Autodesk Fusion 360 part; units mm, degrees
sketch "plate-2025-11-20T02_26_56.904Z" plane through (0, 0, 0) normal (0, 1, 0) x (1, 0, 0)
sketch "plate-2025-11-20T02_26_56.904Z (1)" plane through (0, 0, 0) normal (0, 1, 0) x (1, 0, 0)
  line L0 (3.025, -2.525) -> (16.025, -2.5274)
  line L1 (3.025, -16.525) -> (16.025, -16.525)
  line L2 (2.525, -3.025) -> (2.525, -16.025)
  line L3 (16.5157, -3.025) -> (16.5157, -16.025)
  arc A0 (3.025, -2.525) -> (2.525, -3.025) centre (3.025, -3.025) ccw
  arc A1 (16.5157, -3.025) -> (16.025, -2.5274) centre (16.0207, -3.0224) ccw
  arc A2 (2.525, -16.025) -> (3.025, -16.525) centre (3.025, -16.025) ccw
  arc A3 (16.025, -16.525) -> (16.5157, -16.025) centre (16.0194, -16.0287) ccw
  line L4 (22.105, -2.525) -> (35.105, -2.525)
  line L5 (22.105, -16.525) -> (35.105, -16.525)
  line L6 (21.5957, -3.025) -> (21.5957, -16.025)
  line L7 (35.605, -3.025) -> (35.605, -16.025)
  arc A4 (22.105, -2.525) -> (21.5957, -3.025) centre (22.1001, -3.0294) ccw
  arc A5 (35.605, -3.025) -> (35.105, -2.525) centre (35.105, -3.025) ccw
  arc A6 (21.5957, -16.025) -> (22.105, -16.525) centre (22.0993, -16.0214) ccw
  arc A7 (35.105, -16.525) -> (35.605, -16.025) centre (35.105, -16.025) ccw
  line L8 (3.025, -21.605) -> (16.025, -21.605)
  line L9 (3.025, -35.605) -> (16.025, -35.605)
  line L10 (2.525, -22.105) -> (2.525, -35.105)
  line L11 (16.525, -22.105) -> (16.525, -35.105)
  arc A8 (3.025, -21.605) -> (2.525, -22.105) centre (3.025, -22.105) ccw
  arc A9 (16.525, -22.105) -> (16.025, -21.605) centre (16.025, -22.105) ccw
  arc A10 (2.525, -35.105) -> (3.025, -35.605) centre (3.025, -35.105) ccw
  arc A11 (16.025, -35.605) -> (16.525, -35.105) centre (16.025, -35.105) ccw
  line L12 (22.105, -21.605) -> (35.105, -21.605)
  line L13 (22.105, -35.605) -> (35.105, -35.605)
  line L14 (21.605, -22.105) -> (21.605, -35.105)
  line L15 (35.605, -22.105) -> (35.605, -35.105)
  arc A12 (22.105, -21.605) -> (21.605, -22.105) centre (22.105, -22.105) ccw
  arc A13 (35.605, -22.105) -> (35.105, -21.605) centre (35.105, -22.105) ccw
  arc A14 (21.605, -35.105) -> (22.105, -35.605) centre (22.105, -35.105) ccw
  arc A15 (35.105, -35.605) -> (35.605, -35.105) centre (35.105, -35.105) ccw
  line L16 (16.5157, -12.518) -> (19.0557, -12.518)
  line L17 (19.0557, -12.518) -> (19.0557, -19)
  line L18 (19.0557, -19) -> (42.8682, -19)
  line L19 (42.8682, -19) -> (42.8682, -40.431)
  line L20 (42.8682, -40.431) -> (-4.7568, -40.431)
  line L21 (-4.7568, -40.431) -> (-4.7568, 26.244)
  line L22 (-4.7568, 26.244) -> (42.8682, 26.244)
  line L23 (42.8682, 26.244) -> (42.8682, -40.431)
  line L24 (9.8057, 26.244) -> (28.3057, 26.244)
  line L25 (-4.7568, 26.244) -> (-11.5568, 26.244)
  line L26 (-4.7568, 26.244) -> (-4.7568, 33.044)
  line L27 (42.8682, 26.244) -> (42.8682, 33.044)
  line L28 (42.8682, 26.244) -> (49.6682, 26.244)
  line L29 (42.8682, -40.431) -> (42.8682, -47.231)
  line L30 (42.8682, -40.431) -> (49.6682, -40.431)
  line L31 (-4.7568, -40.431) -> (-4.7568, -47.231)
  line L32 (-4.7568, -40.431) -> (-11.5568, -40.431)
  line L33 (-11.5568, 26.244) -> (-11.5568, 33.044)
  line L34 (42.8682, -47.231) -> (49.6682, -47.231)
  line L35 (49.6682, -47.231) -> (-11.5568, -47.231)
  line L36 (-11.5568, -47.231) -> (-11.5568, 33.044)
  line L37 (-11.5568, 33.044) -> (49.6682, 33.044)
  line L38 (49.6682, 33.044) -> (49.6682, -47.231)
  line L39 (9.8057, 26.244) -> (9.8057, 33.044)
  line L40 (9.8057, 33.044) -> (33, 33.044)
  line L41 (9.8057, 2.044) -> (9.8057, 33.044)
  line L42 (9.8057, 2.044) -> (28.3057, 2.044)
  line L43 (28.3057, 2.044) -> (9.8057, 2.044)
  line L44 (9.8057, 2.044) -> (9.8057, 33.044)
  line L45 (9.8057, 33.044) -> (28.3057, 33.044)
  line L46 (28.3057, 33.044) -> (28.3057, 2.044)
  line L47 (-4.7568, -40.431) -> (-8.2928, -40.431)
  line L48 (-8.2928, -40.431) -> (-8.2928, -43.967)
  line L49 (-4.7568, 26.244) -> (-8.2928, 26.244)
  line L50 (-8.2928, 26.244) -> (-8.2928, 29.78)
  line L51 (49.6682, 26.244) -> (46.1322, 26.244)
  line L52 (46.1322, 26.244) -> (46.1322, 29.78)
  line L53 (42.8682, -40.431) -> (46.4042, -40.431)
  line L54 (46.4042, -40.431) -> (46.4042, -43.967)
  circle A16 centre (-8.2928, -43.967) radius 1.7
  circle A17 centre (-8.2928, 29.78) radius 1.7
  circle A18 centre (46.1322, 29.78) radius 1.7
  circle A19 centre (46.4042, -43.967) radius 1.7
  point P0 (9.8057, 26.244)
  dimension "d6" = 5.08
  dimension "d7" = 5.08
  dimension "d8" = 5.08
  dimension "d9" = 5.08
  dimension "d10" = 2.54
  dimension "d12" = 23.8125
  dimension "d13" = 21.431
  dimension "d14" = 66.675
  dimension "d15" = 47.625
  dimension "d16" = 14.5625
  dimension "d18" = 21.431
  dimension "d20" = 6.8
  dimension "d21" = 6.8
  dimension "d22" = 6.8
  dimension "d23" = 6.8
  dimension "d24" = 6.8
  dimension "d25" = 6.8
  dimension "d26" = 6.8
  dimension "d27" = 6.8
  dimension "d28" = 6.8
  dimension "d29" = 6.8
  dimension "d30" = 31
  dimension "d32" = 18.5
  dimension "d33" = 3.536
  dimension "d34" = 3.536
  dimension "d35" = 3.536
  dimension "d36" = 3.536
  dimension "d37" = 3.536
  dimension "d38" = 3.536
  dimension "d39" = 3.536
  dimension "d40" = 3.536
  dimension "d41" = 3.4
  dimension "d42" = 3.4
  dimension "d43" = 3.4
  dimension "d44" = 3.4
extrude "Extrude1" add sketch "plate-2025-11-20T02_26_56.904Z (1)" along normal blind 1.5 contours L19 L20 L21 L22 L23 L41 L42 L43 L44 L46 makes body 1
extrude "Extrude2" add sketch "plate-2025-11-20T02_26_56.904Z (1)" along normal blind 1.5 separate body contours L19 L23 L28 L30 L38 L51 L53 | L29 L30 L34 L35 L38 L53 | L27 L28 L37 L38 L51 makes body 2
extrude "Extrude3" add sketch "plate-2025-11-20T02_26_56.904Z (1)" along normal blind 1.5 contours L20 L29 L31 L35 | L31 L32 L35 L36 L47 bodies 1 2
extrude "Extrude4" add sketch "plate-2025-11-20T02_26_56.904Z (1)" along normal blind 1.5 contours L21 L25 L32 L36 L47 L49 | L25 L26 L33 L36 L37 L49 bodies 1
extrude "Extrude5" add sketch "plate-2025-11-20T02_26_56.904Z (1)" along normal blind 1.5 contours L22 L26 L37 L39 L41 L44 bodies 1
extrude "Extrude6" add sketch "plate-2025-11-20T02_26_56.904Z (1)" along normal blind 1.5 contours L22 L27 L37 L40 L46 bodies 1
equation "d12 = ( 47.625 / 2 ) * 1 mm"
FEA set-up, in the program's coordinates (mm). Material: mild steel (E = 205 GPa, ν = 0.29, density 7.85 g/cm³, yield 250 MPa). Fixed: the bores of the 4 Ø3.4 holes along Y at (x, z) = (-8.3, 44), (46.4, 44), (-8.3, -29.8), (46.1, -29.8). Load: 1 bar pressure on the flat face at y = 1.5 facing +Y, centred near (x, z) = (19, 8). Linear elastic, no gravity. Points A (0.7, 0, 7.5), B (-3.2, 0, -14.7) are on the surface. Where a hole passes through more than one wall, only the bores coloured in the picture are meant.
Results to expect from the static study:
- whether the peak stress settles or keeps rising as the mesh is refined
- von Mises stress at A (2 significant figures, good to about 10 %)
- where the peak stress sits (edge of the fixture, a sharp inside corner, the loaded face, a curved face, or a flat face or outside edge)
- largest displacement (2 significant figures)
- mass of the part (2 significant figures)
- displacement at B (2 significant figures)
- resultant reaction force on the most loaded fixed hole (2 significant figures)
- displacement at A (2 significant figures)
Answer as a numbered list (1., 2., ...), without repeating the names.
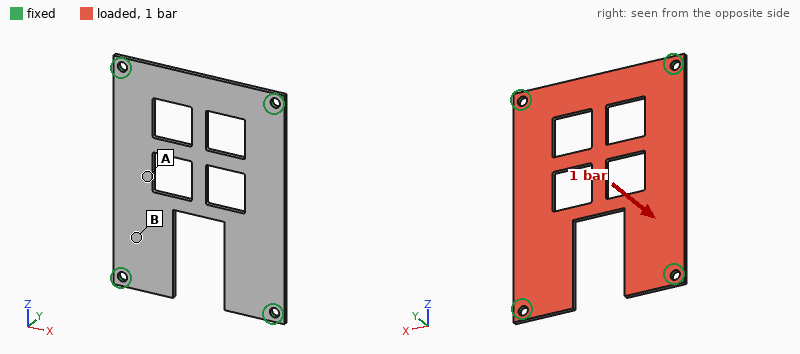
1. keeps rising
2. 81 MPa
3. edge of the fixture
4. 0.24 mm
5. 41 g
6. 0.086 mm
7. 91 N
8. 0.20 mm
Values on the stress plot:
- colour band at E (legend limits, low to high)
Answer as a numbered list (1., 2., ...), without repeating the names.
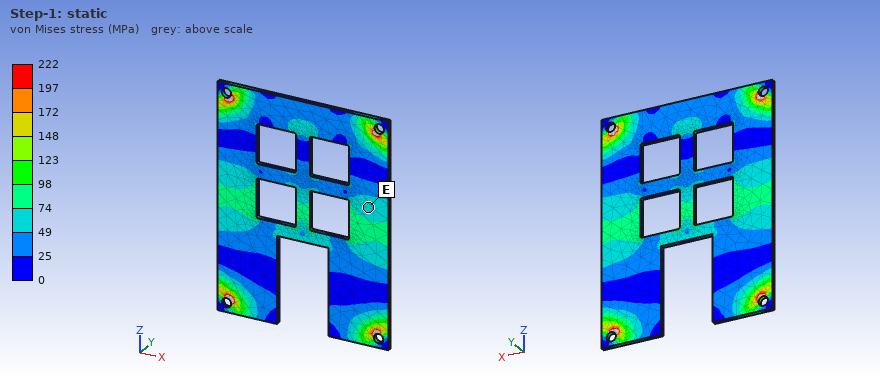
1. 49 to 74 MPa
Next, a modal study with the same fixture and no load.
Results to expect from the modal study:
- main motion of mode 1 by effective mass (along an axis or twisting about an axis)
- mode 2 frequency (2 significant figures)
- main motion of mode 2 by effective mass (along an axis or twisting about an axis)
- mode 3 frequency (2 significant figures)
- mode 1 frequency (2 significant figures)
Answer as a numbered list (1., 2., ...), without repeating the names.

1. along Y
2. 1700 Hz
3. twisting about Z
4. 2500 Hz
5. 1200 Hz
